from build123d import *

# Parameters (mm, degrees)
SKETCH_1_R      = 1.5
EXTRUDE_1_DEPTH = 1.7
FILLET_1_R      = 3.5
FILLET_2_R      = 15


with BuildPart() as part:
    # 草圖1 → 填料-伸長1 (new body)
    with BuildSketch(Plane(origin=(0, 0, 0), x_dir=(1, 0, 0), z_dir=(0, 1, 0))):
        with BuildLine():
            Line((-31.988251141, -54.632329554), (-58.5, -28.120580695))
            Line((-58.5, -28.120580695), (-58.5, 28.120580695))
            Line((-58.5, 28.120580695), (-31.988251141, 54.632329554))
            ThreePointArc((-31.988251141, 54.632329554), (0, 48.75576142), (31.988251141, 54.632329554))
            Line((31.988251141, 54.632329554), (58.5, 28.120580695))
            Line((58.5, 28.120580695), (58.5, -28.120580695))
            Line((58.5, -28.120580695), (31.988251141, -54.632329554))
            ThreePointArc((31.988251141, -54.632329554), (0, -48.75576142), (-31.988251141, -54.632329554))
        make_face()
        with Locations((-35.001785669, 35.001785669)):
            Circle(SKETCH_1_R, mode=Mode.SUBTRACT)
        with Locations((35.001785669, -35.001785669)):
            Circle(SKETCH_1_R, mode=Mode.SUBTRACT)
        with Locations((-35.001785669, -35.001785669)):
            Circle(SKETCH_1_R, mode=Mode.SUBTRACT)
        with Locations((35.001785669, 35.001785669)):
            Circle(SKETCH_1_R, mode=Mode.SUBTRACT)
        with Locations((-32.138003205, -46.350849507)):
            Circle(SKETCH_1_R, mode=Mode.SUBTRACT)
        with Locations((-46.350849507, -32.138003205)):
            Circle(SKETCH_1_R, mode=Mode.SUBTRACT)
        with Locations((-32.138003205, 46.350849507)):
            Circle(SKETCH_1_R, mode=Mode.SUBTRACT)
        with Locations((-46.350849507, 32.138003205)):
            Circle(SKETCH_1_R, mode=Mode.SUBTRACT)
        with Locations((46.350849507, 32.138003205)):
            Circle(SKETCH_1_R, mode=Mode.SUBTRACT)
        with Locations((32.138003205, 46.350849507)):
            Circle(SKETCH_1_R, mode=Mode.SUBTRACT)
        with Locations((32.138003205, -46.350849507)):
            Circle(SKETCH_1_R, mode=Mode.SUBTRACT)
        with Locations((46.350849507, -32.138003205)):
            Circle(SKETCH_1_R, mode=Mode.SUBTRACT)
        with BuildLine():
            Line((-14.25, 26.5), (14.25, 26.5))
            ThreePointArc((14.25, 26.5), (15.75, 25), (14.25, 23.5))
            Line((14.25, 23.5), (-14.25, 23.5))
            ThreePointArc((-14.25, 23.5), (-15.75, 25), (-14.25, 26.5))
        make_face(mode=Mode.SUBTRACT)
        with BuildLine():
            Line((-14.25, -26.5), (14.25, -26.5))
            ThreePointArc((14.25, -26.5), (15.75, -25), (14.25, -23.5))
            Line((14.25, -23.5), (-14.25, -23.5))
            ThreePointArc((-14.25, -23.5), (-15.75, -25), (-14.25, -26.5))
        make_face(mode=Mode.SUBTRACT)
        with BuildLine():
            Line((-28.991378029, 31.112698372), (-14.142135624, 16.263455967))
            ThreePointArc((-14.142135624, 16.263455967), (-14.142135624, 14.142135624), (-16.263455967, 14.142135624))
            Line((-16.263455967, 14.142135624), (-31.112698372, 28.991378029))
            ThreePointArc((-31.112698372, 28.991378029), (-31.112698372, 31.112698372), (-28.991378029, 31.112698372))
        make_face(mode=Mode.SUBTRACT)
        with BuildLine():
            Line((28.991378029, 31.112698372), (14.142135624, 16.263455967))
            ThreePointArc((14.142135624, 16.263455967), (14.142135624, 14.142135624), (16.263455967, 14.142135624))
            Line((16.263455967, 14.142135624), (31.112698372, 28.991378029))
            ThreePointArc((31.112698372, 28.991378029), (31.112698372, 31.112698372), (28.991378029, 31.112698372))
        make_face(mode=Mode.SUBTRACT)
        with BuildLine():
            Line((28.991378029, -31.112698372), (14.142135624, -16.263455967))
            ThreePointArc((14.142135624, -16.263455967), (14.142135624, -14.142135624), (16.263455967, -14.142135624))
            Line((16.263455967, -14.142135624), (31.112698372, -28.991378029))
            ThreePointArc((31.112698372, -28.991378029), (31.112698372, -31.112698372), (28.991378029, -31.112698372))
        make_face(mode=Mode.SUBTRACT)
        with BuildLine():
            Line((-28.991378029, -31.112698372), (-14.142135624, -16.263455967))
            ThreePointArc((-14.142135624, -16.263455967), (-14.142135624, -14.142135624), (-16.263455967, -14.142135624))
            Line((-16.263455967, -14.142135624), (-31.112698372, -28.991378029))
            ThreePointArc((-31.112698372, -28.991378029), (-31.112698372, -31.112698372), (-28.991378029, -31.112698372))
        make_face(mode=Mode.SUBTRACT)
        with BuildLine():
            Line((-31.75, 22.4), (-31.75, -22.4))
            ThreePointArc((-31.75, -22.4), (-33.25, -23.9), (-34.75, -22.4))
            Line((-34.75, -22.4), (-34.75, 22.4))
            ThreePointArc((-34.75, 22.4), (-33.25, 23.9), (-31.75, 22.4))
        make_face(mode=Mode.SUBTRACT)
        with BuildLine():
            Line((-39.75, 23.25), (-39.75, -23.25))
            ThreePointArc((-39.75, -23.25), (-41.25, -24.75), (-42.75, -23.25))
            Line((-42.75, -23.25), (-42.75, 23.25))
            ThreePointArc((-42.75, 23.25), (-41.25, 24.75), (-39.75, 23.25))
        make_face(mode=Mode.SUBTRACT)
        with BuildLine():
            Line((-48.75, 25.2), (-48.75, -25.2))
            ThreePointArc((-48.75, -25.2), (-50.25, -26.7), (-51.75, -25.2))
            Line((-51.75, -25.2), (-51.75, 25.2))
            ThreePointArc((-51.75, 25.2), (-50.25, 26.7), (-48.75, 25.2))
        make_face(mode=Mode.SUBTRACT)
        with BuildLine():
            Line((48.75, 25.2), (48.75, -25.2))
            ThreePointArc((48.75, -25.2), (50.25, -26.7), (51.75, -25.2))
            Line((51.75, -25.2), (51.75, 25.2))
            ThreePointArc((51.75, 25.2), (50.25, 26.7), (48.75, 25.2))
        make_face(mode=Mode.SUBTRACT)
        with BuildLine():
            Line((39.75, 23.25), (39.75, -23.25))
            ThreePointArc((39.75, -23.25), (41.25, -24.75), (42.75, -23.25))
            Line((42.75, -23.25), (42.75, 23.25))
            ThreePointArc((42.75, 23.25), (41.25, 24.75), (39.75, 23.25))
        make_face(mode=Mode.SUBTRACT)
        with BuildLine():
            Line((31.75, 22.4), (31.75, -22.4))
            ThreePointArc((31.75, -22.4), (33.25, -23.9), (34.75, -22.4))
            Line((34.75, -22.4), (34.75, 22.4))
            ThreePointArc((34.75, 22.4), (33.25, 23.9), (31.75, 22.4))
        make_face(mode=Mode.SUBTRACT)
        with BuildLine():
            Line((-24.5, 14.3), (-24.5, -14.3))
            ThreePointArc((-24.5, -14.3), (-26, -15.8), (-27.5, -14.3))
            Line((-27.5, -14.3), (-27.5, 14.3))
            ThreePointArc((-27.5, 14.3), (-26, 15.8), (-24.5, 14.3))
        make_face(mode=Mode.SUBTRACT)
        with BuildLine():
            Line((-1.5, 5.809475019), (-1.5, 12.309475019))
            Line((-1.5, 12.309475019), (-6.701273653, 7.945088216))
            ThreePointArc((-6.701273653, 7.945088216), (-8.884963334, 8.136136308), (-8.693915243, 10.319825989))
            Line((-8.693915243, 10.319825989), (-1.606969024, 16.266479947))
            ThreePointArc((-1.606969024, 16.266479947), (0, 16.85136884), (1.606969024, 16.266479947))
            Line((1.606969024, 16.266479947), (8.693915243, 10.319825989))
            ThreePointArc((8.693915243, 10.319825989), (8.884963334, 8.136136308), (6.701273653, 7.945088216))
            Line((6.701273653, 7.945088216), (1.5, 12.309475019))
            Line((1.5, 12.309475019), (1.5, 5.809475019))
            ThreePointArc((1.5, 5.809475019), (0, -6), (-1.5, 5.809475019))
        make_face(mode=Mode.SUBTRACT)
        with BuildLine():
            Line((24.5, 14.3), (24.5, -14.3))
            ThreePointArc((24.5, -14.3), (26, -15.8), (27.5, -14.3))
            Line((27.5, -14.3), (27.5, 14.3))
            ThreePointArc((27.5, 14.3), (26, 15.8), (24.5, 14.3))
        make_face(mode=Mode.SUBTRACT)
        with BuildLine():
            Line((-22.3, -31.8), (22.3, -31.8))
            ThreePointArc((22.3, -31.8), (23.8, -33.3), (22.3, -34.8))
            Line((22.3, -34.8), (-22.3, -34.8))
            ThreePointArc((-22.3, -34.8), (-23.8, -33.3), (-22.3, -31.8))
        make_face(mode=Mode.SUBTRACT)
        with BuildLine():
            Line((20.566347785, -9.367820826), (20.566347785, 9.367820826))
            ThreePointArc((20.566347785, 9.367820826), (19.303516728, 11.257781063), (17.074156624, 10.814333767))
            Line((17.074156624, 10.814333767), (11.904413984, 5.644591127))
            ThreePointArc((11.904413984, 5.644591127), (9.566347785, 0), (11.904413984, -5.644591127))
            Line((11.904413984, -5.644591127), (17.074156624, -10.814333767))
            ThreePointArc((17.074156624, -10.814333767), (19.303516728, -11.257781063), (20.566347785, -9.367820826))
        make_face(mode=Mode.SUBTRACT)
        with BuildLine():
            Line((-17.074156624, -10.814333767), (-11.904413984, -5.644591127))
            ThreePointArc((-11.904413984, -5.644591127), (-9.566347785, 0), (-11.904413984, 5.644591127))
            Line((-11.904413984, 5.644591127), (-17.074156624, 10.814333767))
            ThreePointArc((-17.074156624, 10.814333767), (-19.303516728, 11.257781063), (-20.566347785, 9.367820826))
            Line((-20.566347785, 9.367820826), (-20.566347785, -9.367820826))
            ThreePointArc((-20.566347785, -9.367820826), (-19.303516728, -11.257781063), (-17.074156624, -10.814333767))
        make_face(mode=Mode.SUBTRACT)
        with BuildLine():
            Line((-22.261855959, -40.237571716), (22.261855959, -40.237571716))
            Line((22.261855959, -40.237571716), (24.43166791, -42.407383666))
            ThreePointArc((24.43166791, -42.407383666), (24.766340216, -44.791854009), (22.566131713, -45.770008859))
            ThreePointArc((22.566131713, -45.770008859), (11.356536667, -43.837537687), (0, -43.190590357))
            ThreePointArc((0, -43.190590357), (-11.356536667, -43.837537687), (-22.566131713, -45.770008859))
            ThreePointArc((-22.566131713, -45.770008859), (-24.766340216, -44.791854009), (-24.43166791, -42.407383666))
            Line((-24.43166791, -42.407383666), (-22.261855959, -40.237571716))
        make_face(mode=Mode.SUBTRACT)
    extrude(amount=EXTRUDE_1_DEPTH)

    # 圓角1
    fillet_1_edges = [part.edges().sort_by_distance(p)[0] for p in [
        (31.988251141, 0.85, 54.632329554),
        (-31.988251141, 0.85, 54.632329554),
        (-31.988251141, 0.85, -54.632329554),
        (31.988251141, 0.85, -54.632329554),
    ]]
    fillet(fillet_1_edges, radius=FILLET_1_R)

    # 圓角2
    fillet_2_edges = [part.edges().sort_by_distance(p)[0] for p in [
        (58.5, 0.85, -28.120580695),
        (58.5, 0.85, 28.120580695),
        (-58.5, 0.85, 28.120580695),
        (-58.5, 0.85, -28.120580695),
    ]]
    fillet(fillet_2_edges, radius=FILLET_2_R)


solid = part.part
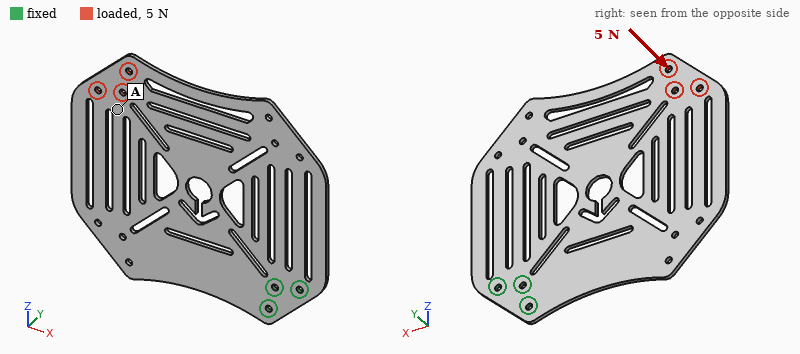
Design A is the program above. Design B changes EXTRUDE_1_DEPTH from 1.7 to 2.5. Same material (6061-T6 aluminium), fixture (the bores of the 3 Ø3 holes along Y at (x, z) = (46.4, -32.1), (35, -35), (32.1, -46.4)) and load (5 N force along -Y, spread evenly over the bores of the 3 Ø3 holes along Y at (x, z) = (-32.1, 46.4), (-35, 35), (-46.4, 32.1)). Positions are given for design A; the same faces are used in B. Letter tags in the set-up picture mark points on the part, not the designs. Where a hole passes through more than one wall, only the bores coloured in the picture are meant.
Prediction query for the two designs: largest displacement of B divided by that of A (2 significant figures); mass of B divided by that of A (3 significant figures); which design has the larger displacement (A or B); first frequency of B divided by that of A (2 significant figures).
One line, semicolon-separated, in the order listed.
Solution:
0.32; 1.47; A; 1.5
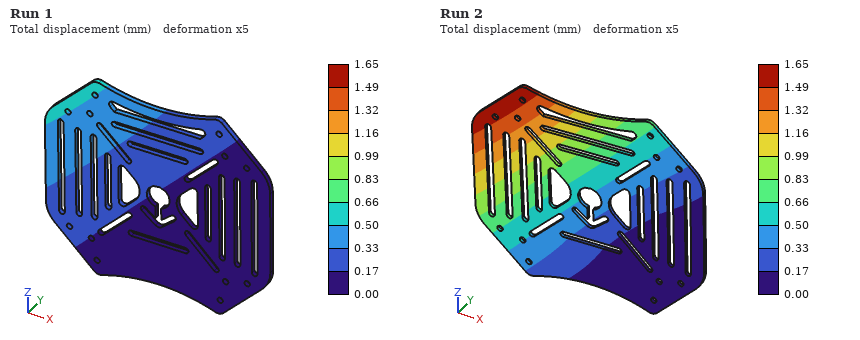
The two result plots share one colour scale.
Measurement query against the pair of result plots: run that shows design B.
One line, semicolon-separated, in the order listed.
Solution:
Run 1
